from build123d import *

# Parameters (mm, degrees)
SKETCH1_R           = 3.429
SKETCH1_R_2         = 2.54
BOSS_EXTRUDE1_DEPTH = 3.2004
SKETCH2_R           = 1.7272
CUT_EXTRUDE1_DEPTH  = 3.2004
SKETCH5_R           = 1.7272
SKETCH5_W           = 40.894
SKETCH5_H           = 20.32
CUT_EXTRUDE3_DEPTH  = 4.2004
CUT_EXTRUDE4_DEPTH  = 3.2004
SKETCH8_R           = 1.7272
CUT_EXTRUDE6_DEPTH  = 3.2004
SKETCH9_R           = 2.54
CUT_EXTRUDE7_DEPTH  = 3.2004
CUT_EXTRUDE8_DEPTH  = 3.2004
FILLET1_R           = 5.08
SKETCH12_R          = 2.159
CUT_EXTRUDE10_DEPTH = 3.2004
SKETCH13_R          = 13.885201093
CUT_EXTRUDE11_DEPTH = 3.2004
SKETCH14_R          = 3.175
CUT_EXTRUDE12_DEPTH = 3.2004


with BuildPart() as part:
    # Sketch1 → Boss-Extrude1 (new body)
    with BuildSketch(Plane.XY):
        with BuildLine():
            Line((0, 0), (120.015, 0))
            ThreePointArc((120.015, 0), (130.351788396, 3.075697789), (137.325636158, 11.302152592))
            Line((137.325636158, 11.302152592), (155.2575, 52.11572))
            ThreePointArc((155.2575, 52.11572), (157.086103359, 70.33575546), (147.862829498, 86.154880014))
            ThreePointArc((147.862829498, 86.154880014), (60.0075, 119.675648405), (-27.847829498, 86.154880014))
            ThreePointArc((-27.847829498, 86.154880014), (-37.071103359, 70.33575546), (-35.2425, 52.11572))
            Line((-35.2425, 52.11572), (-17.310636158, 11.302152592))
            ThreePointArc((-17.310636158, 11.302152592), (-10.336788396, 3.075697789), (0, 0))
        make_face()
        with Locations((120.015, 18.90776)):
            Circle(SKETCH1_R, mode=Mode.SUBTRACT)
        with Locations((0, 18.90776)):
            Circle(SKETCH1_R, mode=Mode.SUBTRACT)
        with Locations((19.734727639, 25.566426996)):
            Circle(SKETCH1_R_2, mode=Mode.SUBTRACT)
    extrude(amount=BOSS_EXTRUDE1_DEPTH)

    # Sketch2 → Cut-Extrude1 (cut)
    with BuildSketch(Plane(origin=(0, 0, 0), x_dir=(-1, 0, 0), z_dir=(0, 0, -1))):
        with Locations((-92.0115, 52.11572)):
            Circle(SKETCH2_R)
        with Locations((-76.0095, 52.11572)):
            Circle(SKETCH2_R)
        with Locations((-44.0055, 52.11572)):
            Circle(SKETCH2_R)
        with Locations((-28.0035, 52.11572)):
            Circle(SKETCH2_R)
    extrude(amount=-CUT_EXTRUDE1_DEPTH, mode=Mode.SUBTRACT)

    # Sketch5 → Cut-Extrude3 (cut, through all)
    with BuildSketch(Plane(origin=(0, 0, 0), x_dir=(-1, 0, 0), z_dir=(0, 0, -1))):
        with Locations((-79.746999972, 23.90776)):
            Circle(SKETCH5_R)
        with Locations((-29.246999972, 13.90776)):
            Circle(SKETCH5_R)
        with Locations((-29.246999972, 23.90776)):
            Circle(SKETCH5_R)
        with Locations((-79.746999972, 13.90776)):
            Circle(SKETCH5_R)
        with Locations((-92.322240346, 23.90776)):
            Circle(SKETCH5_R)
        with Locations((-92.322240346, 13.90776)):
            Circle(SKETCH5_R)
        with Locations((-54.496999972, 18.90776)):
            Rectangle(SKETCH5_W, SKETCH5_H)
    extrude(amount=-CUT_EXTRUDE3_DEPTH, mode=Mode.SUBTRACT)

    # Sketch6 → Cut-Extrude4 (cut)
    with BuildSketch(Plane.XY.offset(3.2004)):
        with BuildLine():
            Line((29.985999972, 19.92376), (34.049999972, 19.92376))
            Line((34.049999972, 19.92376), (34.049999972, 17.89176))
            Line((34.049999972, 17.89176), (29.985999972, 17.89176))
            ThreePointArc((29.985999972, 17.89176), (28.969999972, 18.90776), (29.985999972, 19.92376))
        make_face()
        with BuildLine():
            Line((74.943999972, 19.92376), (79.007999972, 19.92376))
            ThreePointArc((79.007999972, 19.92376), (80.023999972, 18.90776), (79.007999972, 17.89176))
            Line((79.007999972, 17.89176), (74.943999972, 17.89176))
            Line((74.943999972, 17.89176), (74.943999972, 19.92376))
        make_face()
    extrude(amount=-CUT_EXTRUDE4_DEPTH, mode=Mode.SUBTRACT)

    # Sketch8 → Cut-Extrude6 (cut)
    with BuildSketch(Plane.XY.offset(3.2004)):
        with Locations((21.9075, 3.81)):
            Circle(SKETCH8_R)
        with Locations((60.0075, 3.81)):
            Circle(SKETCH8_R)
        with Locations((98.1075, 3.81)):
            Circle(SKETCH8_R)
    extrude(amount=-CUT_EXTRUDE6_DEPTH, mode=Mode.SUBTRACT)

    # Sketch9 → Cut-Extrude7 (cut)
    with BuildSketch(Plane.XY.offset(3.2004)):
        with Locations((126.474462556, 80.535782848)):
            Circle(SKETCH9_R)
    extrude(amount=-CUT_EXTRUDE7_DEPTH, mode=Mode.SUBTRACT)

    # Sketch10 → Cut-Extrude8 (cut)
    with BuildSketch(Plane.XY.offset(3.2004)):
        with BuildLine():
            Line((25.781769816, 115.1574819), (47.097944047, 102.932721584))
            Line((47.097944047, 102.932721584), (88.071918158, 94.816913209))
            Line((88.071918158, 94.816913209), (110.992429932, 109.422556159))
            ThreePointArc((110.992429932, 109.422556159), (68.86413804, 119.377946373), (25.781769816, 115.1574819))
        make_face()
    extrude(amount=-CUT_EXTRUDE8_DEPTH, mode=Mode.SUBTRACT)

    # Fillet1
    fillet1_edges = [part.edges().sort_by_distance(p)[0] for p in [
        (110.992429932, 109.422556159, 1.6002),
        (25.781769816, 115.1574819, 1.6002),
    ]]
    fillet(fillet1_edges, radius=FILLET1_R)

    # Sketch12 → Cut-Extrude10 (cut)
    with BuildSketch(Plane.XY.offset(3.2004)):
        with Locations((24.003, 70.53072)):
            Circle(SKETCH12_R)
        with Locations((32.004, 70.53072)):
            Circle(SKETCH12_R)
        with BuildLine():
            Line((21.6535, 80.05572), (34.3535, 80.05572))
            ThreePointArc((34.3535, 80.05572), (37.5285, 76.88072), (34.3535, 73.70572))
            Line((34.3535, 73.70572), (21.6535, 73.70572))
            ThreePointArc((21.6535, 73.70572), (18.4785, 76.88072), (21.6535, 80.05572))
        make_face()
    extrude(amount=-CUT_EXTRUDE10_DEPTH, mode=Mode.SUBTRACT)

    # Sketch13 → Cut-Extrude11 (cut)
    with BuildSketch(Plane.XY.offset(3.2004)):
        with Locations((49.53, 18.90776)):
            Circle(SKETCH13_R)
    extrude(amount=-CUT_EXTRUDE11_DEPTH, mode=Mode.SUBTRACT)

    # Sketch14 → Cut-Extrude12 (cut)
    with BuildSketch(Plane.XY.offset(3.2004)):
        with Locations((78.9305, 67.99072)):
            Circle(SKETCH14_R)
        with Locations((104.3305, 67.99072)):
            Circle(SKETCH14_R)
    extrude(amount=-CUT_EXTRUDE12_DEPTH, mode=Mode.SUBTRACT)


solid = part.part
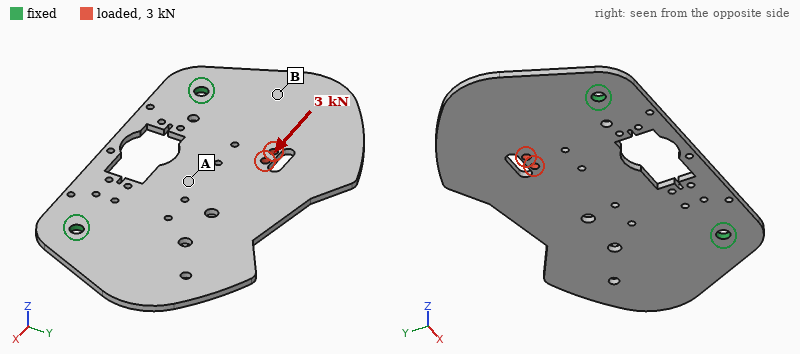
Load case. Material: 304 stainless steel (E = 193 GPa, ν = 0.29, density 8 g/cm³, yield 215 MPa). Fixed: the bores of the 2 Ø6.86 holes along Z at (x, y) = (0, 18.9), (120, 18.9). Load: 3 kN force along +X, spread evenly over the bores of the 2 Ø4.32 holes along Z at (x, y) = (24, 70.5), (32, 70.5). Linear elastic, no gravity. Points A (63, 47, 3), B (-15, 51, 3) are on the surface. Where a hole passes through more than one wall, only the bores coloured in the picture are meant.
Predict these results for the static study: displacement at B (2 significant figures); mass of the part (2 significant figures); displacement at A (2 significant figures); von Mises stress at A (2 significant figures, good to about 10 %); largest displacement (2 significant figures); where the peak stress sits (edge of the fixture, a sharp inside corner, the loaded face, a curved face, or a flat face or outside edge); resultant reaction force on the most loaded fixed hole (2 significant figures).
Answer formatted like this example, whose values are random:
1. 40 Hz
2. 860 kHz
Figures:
1. 7.4 µm
2. 420 g
3. 5.6 µm
4. 16 MPa
5. 14 µm
6. the loaded face
7. 1.9 kN
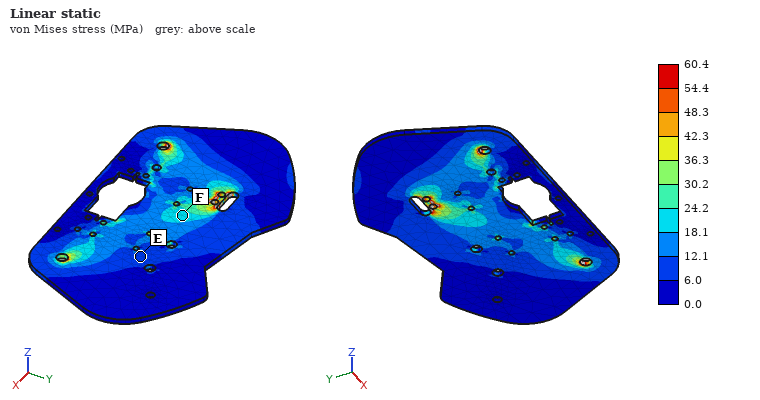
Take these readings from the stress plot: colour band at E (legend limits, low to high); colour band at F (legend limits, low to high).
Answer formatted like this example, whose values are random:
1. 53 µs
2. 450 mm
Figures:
1. 6.0 to 12.1 MPa
2. 18.1 to 24.2 MPa
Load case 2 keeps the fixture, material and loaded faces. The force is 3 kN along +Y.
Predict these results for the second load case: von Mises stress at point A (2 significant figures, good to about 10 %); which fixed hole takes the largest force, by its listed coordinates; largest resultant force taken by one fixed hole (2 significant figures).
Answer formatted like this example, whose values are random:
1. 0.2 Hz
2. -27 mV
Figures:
1. 8.2 MPa
2. (0, 18.9)
3. 2.4 kN
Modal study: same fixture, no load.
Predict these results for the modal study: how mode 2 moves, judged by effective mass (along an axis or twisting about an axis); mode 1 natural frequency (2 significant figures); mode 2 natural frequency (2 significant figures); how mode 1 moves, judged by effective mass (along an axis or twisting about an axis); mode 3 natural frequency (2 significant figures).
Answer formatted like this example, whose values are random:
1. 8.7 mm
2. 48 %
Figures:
1. twisting about Y
2. 290 Hz
3. 510 Hz
4. along Z
5. 810 Hz
